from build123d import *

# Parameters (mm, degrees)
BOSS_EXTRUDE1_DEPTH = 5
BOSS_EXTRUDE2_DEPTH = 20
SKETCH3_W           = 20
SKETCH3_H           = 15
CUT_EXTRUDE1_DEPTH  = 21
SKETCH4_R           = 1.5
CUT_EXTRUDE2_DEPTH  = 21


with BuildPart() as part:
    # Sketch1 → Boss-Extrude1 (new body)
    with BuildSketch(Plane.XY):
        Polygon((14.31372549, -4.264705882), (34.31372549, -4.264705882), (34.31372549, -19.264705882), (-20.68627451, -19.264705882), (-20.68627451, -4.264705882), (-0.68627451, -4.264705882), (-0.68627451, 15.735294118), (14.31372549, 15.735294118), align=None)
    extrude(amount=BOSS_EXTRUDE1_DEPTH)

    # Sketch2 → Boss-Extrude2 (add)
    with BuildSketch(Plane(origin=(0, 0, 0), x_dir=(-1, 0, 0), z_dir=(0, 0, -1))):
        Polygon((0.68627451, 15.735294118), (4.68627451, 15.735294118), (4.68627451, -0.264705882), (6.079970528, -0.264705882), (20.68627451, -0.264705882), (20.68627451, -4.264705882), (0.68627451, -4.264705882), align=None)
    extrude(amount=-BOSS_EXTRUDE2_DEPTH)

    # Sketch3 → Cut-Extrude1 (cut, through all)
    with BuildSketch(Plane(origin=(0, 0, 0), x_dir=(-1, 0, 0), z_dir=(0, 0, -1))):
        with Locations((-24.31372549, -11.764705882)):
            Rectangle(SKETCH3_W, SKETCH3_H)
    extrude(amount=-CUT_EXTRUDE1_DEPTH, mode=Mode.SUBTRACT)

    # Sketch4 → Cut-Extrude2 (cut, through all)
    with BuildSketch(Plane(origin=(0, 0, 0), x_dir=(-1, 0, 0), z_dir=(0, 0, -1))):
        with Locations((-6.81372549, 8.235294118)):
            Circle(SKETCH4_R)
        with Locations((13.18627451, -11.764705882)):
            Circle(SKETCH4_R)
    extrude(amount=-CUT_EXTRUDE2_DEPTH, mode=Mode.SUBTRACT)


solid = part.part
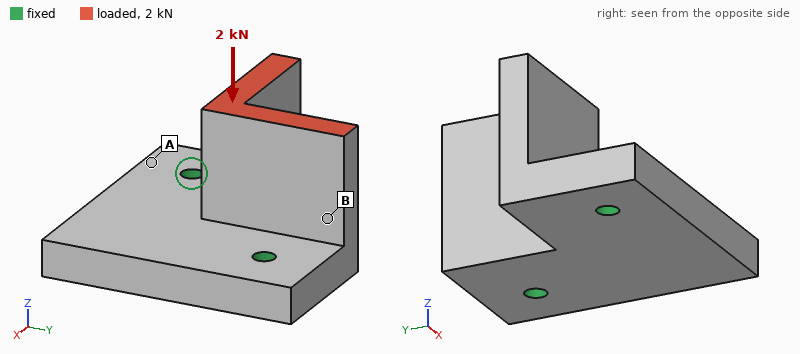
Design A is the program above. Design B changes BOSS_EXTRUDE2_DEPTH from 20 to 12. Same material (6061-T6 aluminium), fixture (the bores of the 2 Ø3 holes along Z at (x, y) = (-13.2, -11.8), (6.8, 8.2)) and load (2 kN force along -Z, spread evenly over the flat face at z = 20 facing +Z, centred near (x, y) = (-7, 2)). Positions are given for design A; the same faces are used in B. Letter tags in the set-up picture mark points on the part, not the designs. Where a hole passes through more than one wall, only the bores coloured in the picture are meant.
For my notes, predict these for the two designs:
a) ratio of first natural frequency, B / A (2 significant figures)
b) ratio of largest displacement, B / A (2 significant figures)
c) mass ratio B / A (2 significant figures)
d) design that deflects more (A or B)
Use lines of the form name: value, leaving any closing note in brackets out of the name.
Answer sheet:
ratio of first natural frequency, B / A: 1.2
ratio of largest displacement, B / A: 0.91
mass ratio B / A: 0.83
design that deflects more: A
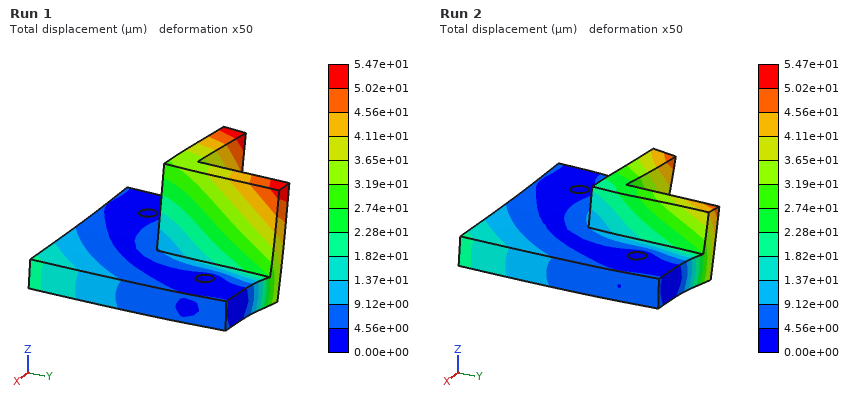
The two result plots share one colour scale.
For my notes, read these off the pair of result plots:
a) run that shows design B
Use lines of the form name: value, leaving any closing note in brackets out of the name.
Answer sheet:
run that shows design B: Run 2
